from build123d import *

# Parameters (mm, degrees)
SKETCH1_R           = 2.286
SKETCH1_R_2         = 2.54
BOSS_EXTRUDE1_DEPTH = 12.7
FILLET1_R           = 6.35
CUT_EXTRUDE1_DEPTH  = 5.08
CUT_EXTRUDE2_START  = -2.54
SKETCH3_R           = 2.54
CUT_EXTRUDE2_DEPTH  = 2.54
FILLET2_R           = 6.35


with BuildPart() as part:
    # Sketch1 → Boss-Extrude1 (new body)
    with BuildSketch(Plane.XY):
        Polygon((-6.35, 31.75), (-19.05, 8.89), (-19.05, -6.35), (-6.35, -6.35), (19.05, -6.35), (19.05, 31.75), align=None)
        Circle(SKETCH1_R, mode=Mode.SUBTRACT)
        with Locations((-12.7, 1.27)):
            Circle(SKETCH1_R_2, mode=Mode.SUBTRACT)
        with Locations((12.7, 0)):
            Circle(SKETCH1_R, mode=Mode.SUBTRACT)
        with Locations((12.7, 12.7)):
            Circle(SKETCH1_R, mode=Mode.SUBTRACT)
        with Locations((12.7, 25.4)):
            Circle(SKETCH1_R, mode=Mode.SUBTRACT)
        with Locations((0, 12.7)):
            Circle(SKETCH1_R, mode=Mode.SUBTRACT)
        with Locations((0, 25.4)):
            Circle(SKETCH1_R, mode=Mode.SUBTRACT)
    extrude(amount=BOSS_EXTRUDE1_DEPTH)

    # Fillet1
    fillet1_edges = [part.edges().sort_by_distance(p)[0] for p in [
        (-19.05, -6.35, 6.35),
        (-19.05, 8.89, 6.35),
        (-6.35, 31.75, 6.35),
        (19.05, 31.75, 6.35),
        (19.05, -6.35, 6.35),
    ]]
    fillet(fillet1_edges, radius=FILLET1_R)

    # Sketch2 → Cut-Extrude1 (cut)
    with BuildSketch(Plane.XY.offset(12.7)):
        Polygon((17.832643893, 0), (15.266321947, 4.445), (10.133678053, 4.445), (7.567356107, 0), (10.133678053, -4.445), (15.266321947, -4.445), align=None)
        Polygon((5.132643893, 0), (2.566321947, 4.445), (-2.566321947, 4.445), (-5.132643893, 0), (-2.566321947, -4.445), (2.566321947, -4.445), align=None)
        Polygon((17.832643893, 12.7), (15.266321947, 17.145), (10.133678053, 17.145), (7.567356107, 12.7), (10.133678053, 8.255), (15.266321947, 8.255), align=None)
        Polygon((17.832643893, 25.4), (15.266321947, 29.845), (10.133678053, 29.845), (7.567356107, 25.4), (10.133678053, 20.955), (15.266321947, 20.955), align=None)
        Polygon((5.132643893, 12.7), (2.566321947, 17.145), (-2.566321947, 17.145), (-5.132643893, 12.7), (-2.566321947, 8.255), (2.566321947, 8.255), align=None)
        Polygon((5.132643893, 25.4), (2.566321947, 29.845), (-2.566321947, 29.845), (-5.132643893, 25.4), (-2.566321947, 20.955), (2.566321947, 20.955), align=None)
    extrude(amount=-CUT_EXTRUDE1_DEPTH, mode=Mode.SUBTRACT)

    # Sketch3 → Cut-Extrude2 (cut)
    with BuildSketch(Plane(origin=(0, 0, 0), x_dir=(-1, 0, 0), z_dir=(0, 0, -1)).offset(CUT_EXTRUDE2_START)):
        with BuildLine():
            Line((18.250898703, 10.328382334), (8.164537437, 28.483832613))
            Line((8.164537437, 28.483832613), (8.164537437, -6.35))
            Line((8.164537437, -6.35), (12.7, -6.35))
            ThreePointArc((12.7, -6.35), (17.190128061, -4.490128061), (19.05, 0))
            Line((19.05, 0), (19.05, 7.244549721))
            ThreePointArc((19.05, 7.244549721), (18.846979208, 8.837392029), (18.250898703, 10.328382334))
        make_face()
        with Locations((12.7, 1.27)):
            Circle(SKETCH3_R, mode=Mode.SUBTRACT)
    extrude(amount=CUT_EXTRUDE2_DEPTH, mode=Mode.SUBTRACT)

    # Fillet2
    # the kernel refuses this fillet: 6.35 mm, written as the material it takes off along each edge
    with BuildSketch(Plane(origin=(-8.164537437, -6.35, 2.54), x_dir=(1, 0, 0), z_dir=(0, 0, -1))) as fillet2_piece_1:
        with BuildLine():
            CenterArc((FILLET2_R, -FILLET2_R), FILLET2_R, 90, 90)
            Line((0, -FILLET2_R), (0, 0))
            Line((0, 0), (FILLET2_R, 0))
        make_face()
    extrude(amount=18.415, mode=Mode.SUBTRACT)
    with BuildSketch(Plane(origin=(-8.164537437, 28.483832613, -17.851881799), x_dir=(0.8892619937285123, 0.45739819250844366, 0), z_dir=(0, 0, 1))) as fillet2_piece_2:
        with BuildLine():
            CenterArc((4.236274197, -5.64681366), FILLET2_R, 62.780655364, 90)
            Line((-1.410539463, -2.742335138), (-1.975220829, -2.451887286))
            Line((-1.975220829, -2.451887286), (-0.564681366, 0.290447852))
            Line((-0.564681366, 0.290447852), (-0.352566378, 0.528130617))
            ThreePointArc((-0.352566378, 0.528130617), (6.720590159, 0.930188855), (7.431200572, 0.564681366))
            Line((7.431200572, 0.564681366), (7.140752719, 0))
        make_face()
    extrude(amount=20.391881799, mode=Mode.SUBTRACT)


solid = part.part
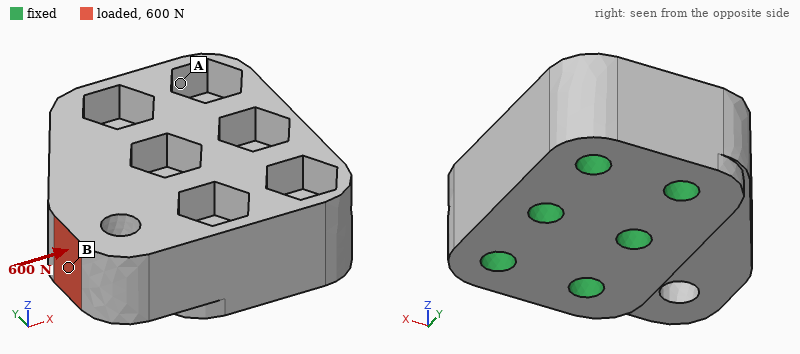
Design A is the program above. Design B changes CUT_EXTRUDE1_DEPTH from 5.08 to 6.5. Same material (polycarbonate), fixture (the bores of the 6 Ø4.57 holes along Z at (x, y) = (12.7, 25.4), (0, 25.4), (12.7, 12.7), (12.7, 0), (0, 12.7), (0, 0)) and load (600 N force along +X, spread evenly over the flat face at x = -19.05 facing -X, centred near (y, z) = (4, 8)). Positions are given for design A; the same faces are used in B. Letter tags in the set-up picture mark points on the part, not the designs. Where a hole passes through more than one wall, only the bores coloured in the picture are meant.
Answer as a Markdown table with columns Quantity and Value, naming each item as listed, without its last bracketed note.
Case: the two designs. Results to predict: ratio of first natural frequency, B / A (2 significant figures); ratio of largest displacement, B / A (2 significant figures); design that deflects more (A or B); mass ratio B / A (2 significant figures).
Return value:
| Quantity | Value |
|---|---|
| ratio of first natural frequency, B / A | 0.91 |
| ratio of largest displacement, B / A | 1.2 |
| design that deflects more | B |
| mass ratio B / A | 0.96 |
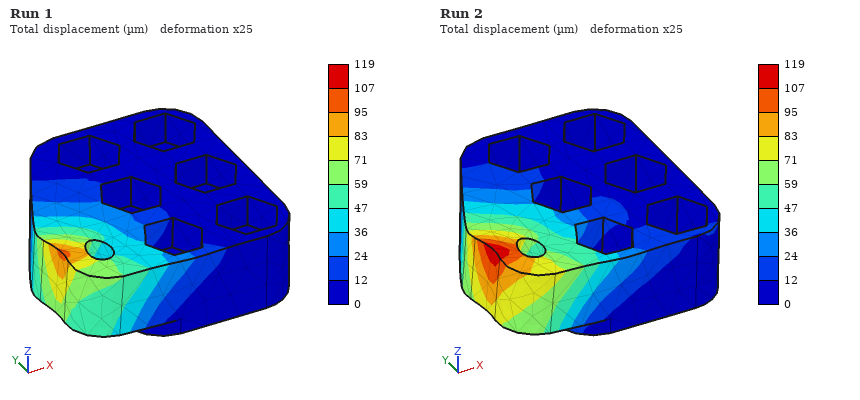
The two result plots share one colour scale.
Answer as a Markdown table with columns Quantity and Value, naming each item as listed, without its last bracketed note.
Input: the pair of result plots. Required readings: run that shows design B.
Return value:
| Quantity | Value |
|---|---|
| run that shows design B | Run 2 |
